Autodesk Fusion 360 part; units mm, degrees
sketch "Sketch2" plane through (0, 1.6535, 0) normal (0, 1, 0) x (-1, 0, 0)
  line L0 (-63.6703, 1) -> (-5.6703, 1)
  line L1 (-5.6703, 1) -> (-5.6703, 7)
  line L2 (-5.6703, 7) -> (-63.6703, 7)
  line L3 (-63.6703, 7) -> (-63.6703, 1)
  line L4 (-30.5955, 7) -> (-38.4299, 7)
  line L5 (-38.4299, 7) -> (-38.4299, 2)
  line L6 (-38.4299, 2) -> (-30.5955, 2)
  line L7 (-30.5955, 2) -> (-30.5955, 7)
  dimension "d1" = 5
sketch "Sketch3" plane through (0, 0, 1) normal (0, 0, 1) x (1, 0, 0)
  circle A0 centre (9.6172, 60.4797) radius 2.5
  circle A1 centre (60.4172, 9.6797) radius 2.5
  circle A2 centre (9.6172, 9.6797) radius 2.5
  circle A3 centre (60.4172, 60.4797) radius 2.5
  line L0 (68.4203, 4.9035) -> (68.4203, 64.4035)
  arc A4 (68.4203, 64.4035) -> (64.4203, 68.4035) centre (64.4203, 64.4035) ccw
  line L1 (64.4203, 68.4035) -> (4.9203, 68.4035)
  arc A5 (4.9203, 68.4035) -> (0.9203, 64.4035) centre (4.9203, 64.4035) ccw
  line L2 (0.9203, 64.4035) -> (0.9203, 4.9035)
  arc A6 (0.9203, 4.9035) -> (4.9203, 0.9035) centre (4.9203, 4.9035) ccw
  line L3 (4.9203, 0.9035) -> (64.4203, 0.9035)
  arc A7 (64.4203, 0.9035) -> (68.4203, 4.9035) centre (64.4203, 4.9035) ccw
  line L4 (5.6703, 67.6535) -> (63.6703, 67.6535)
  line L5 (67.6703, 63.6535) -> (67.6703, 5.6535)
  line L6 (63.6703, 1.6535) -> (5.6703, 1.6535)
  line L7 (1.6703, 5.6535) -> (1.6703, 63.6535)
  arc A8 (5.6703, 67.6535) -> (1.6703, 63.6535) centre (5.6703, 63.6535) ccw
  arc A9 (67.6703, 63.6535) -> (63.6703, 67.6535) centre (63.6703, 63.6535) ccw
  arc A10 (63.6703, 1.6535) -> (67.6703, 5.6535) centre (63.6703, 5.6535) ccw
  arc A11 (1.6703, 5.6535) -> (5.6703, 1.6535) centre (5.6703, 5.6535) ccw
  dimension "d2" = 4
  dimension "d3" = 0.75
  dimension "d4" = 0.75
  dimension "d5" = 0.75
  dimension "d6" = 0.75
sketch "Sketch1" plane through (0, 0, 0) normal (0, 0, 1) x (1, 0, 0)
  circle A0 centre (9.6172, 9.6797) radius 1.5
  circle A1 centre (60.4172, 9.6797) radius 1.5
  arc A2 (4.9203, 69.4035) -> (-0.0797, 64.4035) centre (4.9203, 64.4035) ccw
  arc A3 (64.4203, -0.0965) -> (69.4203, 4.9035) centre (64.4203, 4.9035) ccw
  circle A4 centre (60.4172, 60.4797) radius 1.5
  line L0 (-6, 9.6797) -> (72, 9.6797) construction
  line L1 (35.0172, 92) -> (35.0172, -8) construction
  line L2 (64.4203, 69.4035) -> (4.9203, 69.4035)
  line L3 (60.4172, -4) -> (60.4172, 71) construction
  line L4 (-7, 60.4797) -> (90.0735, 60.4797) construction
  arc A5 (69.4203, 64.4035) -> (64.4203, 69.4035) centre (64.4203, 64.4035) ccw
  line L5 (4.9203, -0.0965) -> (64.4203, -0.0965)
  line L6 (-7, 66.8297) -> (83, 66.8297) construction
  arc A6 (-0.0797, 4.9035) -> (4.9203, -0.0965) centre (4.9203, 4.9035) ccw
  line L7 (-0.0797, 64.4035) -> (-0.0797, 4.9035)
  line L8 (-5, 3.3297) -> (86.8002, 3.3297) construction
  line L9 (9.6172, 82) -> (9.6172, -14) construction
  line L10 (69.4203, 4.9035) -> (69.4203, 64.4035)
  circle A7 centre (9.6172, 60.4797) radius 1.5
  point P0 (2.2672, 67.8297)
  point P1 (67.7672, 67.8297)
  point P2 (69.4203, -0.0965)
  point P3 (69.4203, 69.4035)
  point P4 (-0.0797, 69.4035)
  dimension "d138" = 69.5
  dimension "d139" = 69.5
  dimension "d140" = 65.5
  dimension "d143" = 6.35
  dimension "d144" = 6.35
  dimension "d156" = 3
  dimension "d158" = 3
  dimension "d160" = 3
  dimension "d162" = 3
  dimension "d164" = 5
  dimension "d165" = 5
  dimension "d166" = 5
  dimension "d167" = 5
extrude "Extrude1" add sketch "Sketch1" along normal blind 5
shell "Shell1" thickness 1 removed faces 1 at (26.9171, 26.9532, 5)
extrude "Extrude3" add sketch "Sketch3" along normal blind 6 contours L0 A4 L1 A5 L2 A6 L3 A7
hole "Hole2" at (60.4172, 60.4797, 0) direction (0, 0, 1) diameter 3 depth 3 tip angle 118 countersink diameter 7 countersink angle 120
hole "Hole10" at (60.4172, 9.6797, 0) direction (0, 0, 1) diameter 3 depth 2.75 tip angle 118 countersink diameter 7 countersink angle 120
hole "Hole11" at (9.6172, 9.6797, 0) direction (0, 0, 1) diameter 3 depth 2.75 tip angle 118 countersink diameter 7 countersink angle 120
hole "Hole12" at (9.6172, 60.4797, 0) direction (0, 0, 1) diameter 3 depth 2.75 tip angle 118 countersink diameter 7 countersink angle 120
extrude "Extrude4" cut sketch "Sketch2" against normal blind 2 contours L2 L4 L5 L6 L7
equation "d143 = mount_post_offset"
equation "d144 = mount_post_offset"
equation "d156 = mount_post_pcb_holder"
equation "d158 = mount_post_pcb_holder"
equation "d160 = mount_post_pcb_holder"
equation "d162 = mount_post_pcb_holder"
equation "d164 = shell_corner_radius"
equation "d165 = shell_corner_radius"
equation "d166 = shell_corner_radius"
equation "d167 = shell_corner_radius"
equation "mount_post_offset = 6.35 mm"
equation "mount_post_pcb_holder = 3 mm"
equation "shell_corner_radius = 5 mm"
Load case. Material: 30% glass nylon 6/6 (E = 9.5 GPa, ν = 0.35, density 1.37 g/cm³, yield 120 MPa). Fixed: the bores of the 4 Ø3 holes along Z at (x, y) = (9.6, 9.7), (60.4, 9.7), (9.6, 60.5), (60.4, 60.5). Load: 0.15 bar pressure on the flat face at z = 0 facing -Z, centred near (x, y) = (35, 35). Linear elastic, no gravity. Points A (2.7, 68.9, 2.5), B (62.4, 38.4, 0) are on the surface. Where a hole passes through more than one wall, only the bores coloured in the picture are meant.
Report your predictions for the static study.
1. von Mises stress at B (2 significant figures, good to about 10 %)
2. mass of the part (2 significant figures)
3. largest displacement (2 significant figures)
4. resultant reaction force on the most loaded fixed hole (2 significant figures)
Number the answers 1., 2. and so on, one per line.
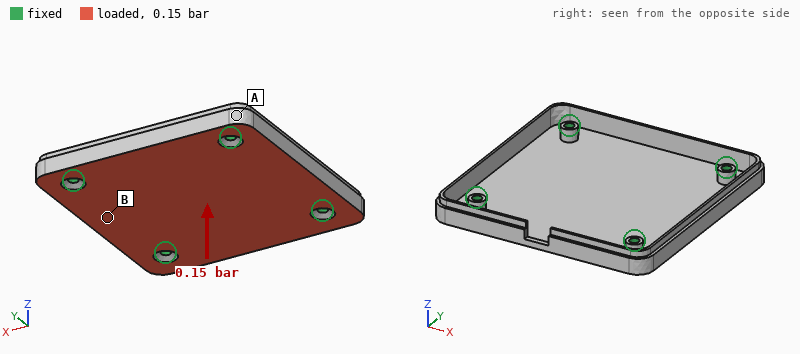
1. 4.7 MPa
2. 9.8 g
3. 0.59 mm
4. 32 N
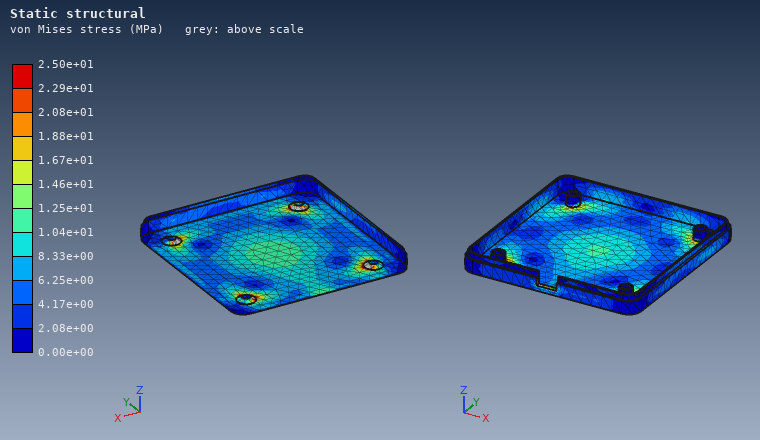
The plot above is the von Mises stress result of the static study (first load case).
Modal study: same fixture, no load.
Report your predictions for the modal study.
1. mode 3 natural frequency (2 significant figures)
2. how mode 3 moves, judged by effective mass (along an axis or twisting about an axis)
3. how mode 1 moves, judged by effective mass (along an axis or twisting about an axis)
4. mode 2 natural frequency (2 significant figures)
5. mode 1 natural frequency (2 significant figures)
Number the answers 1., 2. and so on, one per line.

1. 1800 Hz
2. twisting about Y
3. along Z
4. 1300 Hz
5. 850 Hz
